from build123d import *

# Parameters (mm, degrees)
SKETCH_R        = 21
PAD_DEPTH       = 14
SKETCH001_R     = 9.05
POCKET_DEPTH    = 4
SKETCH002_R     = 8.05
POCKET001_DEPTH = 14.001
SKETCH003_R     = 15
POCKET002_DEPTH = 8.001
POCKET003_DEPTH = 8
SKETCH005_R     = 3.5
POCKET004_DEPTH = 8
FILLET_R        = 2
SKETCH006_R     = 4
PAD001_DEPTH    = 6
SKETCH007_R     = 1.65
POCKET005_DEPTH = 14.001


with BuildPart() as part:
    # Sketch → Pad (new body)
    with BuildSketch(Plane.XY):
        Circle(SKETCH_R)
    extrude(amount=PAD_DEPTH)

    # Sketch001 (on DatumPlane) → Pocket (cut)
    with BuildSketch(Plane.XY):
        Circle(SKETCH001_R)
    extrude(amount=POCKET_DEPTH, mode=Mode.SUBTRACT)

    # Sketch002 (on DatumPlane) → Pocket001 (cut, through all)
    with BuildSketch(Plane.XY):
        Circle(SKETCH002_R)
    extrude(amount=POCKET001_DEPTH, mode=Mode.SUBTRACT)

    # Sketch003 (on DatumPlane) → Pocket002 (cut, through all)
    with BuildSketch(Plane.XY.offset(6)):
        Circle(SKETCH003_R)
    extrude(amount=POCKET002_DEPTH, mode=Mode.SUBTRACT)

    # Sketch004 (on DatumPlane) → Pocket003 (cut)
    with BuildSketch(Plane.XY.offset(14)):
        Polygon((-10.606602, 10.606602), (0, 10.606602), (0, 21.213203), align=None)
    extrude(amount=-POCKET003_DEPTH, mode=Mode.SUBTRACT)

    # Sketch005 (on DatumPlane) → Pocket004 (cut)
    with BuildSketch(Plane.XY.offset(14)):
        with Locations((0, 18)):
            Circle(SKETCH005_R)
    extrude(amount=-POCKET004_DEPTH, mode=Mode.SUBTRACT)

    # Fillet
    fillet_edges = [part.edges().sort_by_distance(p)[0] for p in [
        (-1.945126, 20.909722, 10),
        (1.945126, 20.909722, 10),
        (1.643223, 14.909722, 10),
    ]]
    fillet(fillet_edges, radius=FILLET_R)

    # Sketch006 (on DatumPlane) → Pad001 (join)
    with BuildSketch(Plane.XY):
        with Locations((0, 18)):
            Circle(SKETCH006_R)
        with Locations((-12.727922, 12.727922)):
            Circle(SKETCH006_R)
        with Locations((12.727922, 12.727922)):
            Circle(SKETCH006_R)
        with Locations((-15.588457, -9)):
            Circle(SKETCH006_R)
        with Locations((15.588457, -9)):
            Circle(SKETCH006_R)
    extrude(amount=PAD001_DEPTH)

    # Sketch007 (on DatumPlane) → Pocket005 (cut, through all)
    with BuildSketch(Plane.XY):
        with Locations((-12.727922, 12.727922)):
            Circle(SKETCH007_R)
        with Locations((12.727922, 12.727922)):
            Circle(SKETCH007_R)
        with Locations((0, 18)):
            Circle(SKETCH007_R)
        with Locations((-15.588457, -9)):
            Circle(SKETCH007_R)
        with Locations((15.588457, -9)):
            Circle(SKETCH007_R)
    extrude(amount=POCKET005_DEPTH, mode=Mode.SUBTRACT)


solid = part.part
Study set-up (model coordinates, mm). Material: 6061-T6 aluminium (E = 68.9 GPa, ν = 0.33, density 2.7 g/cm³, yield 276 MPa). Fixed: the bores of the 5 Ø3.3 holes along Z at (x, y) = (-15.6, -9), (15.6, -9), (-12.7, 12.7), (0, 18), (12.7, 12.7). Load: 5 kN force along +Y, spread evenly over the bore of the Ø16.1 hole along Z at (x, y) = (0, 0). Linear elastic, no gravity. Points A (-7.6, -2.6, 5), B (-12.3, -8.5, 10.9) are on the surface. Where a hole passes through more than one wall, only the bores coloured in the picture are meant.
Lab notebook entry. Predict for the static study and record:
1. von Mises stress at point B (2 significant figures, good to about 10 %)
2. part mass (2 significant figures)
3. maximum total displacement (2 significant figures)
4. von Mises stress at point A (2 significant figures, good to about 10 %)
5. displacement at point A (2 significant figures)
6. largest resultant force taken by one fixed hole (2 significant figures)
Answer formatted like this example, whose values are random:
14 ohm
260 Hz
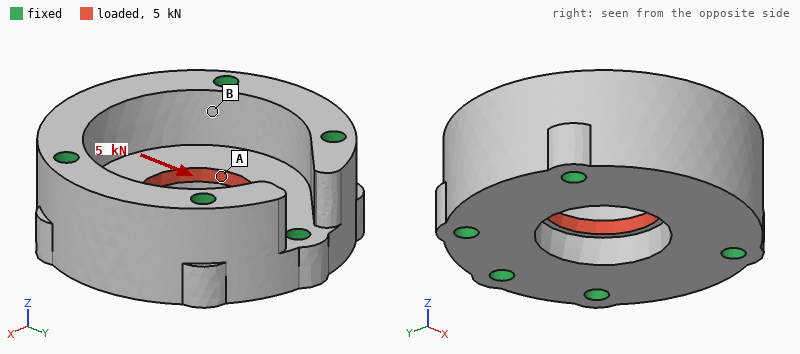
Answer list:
10 MPa
31 g
9.3 µm
80 MPa
6.3 µm
1.2 kN
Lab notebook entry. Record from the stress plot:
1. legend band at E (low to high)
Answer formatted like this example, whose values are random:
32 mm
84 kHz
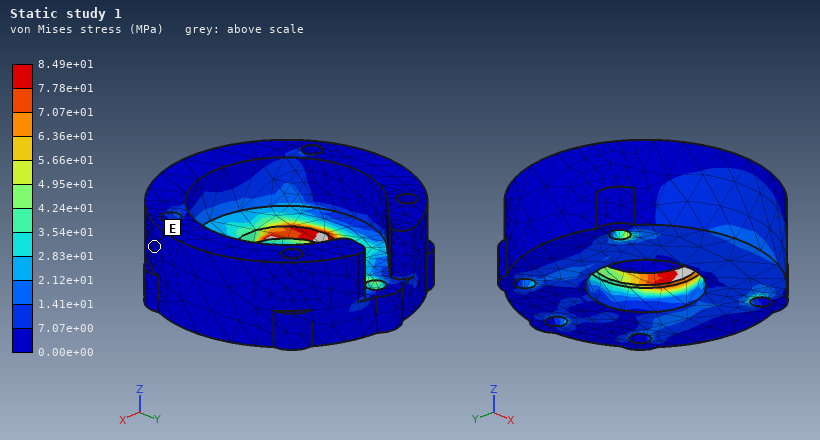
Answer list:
0.00e+00 to 7.07e+00 MPa
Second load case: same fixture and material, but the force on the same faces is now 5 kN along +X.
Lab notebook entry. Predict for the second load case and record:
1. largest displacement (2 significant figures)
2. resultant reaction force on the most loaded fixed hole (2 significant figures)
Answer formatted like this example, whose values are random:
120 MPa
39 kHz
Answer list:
7.4 µm
1.4 kN
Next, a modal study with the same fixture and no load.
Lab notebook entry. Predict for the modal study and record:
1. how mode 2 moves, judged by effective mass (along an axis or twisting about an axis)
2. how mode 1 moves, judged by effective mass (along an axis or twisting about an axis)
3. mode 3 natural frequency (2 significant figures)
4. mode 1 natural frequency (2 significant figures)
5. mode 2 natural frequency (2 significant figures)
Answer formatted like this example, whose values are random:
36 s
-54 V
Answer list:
along Y
along Z
46 kHz
30 kHz
42 kHz
